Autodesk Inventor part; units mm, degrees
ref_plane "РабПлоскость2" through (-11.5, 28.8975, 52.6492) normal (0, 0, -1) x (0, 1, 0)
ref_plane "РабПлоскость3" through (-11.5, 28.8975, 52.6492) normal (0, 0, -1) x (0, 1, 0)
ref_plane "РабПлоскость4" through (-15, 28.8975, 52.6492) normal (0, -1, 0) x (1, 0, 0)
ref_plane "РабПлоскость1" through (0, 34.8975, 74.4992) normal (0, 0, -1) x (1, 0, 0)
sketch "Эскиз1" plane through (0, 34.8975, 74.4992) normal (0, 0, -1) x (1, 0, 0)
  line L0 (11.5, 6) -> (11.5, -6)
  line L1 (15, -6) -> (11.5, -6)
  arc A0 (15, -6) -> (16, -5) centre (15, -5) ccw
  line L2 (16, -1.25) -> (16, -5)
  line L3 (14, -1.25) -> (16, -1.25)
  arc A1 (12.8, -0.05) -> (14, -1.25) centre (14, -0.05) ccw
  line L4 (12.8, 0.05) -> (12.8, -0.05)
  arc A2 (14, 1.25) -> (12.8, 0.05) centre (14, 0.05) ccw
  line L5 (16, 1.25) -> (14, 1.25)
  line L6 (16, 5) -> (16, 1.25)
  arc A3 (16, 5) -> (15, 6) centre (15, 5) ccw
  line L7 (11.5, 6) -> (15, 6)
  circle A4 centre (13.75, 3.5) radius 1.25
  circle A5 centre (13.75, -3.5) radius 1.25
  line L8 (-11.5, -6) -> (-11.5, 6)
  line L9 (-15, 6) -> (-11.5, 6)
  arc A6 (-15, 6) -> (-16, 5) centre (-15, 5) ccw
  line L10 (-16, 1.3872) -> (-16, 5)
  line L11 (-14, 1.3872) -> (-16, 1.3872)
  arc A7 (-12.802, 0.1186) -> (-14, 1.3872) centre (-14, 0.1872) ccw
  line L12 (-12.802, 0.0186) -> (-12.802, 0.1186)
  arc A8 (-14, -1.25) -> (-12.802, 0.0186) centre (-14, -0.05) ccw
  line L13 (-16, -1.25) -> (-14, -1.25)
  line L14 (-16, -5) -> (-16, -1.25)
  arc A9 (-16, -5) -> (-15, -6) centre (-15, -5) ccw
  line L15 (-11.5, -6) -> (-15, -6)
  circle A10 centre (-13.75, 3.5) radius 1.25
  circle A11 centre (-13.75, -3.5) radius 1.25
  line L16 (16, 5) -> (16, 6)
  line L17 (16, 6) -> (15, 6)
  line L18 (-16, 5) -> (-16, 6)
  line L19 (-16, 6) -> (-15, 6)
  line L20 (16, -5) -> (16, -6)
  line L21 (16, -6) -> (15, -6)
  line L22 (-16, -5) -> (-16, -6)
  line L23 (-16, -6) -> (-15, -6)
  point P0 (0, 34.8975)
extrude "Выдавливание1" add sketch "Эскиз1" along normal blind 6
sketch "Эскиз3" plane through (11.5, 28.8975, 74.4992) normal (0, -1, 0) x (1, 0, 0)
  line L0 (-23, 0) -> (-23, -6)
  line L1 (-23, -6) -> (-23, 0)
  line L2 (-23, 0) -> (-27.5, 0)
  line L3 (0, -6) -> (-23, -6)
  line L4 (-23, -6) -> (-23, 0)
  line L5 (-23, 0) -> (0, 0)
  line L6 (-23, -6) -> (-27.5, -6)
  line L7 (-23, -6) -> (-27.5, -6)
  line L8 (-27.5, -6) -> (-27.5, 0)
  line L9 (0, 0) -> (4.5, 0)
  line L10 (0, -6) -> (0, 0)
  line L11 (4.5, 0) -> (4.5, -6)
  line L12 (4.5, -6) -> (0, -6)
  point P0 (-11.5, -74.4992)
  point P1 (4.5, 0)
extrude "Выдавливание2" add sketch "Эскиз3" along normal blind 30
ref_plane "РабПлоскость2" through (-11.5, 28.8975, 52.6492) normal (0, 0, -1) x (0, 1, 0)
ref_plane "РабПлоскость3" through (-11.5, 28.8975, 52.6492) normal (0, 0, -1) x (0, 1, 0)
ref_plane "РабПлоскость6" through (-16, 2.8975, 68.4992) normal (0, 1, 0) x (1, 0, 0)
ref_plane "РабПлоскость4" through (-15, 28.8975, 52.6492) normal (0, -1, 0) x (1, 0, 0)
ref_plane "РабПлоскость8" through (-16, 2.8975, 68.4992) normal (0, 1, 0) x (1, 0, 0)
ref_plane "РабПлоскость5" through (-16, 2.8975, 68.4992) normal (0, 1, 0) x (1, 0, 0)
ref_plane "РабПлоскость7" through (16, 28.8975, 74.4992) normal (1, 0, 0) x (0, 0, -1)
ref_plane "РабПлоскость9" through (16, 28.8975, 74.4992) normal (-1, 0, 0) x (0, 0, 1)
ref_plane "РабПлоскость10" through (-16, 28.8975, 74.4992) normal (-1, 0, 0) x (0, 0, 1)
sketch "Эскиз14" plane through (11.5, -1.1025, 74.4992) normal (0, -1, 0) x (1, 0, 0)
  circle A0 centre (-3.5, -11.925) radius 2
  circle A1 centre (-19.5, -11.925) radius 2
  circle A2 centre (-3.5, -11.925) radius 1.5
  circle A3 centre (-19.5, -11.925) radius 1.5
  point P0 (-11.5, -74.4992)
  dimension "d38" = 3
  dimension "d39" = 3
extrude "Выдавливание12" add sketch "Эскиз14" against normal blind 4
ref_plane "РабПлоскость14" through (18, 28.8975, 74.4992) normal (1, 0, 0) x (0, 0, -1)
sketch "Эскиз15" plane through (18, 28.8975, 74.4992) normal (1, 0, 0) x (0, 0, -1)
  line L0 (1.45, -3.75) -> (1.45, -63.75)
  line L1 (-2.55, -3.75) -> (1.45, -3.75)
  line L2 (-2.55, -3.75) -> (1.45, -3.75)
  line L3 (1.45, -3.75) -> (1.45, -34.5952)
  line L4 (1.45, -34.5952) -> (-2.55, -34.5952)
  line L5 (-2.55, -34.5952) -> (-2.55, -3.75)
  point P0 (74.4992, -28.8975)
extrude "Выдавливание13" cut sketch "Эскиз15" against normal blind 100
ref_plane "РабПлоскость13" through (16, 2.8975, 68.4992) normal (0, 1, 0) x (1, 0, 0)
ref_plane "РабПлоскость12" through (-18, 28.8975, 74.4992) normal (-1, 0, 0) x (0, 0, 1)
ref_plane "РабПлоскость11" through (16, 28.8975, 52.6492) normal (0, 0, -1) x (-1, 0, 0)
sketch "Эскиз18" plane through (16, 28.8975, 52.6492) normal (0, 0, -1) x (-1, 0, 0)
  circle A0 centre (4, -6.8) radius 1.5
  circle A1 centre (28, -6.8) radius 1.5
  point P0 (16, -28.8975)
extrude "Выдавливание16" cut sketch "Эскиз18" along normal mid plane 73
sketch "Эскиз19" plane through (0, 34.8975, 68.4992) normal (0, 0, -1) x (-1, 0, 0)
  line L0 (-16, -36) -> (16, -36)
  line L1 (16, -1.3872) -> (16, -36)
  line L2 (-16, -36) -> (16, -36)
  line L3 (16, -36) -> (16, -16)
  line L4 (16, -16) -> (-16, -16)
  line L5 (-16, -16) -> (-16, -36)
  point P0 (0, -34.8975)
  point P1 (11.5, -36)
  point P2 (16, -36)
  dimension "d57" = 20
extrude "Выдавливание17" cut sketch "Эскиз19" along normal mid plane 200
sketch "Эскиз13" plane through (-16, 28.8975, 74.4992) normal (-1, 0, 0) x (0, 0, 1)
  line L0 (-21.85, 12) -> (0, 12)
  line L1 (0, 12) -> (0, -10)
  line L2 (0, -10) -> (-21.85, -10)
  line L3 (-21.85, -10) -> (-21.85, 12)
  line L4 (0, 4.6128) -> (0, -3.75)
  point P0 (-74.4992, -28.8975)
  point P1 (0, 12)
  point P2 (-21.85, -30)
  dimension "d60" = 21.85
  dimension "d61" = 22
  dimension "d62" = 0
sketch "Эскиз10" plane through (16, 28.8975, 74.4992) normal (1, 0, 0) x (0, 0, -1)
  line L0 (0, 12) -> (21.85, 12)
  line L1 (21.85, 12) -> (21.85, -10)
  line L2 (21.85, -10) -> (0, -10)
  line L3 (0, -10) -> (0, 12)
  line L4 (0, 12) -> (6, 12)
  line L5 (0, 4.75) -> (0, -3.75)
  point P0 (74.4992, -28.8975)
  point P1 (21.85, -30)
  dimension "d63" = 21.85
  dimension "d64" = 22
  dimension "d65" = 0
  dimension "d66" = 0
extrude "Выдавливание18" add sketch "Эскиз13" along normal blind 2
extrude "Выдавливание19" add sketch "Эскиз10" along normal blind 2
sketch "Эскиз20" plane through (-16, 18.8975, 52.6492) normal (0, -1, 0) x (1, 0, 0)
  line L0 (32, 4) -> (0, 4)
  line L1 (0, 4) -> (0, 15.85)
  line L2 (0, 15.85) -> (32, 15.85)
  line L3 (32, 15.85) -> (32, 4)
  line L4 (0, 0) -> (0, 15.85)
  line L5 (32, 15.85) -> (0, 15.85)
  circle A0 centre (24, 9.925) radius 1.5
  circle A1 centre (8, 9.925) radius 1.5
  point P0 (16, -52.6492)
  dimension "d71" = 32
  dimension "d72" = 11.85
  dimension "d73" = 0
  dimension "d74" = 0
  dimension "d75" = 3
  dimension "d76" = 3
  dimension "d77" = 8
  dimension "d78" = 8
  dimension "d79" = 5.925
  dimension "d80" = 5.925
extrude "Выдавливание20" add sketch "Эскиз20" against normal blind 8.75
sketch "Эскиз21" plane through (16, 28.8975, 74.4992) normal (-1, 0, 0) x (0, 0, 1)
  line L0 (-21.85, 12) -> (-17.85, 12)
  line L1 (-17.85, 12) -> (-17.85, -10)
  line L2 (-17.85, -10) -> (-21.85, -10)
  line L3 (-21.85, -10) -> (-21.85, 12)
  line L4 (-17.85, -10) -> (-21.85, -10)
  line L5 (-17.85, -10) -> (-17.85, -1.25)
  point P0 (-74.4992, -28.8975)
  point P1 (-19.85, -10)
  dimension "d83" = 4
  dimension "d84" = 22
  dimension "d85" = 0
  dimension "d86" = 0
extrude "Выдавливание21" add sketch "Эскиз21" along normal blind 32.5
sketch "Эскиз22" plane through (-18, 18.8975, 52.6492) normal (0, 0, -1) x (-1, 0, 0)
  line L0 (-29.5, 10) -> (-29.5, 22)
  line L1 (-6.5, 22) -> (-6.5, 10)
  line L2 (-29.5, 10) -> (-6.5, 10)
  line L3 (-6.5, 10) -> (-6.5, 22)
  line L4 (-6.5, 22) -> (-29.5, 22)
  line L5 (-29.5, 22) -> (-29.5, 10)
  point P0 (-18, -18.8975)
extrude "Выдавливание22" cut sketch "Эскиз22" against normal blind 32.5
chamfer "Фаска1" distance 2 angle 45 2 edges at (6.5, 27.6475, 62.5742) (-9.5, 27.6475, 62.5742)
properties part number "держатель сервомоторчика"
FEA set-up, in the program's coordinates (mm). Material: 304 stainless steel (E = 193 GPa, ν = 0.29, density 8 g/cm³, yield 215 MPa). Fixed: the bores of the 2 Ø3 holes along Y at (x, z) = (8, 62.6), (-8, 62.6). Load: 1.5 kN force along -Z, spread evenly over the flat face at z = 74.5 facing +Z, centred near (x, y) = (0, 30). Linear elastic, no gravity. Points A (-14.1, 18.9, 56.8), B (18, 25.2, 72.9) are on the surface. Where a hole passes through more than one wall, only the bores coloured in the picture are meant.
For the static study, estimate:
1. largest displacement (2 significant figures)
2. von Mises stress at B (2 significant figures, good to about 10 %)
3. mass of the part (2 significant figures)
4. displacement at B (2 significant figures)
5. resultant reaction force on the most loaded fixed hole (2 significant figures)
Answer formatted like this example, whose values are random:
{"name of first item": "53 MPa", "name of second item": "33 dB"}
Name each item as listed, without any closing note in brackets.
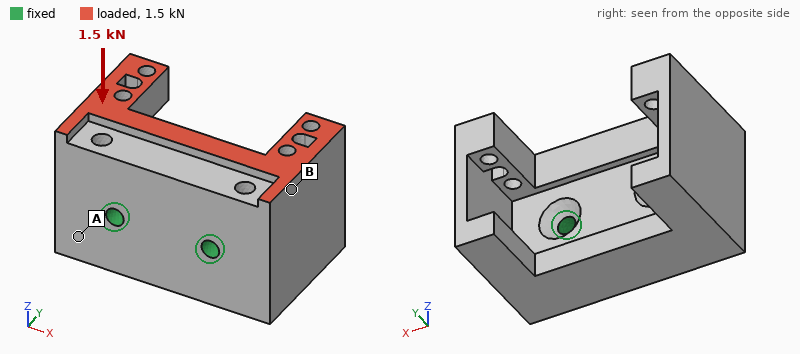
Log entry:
{"largest displacement": "10 µm", "von Mises stress at B": "13 MPa", "mass of the part": "70 g", "displacement at B": "3.6 µm", "resultant reaction force on the most loaded fixed hole": "750 N"}
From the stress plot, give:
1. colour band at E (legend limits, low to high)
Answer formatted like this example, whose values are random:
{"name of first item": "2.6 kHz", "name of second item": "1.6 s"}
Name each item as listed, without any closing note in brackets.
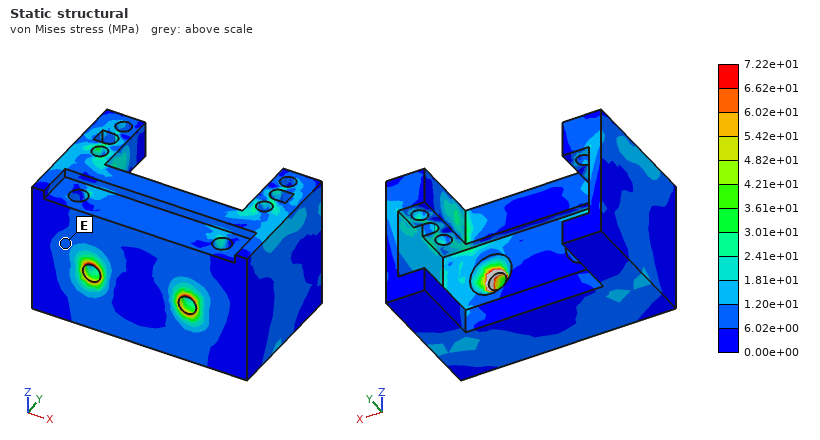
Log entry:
{"colour band at E": "6.02e+00 to 1.20e+01 MPa"}
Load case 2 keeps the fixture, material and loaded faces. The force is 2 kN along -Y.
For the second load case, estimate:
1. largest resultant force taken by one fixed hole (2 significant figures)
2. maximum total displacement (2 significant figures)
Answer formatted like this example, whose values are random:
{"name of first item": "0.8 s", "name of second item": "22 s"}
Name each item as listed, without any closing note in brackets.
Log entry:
{"largest resultant force taken by one fixed hole": "1.0 kN", "maximum total displacement": "18 µm"}
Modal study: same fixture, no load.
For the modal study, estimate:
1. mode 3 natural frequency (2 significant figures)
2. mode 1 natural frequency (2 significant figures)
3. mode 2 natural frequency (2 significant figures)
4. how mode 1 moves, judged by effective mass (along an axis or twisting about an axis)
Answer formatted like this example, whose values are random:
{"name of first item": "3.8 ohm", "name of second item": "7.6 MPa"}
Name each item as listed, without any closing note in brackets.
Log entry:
{"mode 3 natural frequency": "14 kHz", "mode 1 natural frequency": "13 kHz", "mode 2 natural frequency": "14 kHz", "how mode 1 moves, judged by effective mass": "along Z"}
